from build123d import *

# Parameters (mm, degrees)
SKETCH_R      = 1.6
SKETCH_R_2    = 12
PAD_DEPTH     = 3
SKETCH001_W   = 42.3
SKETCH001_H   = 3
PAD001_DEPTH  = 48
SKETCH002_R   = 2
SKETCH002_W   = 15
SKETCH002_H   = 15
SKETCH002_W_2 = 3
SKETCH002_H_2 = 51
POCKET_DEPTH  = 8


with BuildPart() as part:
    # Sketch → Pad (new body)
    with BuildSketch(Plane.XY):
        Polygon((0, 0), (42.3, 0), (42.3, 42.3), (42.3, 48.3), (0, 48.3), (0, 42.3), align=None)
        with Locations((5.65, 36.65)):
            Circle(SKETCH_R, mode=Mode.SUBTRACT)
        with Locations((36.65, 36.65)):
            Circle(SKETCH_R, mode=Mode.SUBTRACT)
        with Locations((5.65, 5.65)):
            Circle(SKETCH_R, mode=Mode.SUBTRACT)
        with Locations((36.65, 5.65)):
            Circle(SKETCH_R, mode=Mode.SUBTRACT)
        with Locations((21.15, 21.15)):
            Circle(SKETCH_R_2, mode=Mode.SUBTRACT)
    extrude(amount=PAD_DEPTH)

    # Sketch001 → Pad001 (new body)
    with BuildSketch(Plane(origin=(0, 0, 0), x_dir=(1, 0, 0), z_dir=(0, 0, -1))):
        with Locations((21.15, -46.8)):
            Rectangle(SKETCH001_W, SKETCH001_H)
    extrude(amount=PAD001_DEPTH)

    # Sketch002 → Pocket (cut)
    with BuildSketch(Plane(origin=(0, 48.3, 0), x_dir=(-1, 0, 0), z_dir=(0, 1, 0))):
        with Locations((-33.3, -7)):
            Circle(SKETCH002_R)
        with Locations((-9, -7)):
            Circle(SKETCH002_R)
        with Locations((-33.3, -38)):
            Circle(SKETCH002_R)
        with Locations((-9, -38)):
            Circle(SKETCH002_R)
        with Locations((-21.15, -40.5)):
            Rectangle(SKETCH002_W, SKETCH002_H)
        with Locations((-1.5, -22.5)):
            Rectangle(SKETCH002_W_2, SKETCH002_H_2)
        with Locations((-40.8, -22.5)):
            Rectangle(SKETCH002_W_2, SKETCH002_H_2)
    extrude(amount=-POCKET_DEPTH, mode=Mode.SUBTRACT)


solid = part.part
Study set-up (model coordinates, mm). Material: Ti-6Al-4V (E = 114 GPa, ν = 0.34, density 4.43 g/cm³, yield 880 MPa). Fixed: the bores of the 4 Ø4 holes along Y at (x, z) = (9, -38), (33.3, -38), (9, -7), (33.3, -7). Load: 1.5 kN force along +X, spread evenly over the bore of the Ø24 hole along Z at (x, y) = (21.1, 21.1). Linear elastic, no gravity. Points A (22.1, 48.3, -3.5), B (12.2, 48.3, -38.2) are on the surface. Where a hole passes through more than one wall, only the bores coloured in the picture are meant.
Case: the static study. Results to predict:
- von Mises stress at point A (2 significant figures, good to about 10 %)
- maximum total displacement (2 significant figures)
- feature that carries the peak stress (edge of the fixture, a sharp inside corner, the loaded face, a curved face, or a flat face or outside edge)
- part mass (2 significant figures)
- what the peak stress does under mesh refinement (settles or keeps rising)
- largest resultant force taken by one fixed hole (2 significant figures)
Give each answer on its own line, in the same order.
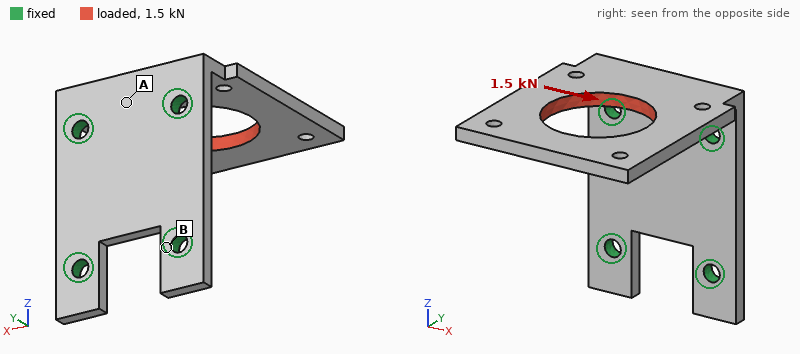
52 MPa
0.26 mm
edge of the fixture
40 g
keeps rising
1.7 kN
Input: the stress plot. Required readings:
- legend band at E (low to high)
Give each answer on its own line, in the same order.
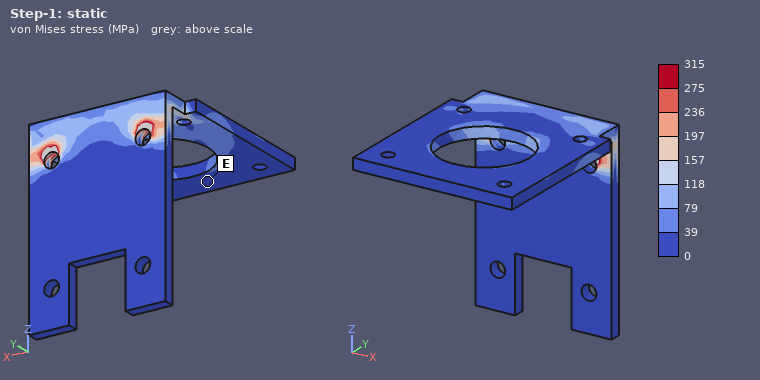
0 to 39 MPa
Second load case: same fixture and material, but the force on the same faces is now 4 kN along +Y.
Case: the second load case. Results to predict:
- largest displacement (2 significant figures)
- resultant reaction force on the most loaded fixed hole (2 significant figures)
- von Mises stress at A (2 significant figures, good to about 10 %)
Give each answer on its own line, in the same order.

0.65 mm
2.1 kN
170 MPa
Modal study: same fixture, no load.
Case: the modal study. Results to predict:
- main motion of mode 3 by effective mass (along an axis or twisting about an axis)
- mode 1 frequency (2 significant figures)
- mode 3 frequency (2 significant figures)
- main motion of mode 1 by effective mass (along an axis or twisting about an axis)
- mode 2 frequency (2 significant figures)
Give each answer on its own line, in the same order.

along X
870 Hz
3600 Hz
along Z
2200 Hz
